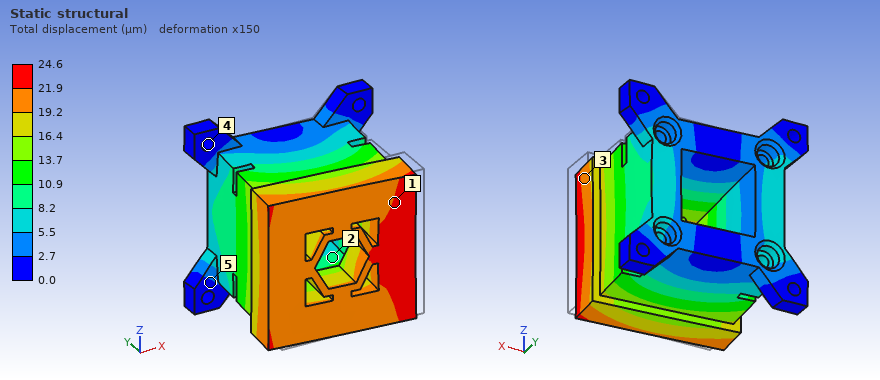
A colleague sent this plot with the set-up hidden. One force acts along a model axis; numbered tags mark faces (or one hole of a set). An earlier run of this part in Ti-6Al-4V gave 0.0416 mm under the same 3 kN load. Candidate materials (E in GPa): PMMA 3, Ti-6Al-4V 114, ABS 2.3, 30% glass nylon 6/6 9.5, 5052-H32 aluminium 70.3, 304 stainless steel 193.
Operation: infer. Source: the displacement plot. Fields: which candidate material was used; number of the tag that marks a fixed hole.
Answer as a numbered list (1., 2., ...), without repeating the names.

1. 304 stainless steel
2. 4
